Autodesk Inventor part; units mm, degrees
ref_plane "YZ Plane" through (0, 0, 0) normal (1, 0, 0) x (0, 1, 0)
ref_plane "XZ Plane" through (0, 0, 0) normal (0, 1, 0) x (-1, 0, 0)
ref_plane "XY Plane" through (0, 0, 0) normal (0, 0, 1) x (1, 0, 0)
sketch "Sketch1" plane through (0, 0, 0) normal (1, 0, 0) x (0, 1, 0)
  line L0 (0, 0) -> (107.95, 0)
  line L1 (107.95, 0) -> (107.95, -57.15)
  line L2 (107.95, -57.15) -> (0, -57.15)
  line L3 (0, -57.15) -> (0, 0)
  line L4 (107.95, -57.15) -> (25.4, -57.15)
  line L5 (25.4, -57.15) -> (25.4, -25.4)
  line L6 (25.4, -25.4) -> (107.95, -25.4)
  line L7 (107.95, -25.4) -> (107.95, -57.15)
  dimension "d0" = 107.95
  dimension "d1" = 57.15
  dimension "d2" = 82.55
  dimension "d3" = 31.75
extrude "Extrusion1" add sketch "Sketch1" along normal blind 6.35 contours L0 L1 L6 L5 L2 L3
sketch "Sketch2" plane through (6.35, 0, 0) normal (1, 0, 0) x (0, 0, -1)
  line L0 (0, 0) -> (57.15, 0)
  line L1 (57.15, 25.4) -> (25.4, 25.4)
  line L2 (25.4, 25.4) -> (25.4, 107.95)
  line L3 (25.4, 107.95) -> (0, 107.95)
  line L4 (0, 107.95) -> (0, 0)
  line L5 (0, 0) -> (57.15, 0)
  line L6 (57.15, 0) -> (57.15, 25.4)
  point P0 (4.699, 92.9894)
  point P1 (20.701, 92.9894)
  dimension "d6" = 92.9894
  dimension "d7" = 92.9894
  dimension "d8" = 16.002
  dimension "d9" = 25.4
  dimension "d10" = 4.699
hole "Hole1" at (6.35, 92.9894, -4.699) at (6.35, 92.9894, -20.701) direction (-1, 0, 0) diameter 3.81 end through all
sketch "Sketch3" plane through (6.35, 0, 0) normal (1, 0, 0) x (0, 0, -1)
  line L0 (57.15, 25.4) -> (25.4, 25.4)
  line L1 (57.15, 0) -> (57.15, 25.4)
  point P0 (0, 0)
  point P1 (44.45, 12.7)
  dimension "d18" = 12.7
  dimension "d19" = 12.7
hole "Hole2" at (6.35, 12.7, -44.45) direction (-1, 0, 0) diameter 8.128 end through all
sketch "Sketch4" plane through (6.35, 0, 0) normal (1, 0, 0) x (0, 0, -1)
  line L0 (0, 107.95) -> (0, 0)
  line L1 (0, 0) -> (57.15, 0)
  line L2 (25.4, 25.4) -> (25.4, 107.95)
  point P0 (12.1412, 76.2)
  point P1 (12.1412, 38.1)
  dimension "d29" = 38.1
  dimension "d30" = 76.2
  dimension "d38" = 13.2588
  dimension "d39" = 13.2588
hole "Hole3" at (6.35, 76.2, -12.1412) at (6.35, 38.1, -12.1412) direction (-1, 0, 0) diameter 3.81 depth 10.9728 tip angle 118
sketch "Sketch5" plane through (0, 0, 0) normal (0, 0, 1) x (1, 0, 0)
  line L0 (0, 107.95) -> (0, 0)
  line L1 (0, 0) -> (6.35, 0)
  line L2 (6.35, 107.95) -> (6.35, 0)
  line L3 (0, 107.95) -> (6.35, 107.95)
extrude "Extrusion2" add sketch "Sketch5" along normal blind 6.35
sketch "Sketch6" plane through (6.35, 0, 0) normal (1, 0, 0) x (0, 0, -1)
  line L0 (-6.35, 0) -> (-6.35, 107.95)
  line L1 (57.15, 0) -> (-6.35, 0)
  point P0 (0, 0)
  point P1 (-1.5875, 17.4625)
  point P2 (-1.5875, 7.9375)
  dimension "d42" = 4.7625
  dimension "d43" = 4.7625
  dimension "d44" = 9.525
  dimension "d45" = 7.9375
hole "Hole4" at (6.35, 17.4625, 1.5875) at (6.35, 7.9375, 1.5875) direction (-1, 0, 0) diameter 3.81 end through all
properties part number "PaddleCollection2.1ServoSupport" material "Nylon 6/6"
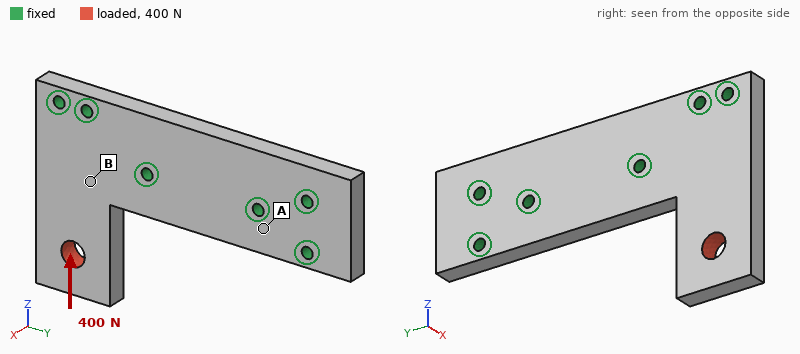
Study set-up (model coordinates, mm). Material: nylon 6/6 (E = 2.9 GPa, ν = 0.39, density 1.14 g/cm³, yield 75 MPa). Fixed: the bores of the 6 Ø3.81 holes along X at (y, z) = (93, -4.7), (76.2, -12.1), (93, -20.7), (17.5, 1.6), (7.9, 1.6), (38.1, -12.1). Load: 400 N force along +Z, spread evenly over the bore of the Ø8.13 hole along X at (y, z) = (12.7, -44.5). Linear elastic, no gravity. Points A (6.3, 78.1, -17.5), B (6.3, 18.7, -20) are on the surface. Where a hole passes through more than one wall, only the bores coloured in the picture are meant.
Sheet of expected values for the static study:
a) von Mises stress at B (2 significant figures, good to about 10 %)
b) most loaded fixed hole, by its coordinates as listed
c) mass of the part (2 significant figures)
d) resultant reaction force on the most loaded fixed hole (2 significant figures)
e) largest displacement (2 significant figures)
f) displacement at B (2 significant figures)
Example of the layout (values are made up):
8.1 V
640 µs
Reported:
2.3 MPa
(7.9, 1.6)
30 g
220 N
58 µm
16 µm
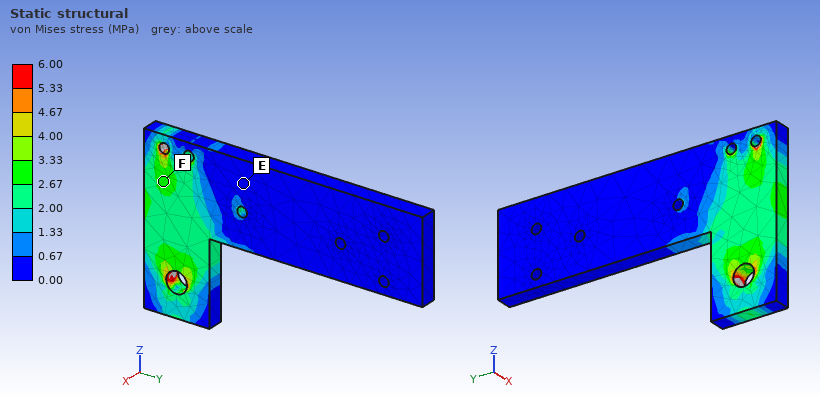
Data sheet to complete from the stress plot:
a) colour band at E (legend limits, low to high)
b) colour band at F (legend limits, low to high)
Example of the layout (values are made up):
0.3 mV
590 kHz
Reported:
0.00 to 0.67 MPa
2.67 to 3.33 MPa
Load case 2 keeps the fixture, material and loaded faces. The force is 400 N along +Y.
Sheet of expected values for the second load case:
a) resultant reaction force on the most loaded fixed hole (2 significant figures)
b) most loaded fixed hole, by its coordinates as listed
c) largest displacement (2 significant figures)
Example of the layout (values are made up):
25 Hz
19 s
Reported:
490 N
(38.1, -12.1)
0.39 mm
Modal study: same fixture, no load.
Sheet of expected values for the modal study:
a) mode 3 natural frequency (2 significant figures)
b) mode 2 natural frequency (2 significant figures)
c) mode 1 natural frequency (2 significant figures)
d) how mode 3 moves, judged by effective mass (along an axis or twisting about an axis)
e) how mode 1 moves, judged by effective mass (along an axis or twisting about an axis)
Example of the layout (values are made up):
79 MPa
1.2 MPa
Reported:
2700 Hz
2400 Hz
660 Hz
along Y
along X
